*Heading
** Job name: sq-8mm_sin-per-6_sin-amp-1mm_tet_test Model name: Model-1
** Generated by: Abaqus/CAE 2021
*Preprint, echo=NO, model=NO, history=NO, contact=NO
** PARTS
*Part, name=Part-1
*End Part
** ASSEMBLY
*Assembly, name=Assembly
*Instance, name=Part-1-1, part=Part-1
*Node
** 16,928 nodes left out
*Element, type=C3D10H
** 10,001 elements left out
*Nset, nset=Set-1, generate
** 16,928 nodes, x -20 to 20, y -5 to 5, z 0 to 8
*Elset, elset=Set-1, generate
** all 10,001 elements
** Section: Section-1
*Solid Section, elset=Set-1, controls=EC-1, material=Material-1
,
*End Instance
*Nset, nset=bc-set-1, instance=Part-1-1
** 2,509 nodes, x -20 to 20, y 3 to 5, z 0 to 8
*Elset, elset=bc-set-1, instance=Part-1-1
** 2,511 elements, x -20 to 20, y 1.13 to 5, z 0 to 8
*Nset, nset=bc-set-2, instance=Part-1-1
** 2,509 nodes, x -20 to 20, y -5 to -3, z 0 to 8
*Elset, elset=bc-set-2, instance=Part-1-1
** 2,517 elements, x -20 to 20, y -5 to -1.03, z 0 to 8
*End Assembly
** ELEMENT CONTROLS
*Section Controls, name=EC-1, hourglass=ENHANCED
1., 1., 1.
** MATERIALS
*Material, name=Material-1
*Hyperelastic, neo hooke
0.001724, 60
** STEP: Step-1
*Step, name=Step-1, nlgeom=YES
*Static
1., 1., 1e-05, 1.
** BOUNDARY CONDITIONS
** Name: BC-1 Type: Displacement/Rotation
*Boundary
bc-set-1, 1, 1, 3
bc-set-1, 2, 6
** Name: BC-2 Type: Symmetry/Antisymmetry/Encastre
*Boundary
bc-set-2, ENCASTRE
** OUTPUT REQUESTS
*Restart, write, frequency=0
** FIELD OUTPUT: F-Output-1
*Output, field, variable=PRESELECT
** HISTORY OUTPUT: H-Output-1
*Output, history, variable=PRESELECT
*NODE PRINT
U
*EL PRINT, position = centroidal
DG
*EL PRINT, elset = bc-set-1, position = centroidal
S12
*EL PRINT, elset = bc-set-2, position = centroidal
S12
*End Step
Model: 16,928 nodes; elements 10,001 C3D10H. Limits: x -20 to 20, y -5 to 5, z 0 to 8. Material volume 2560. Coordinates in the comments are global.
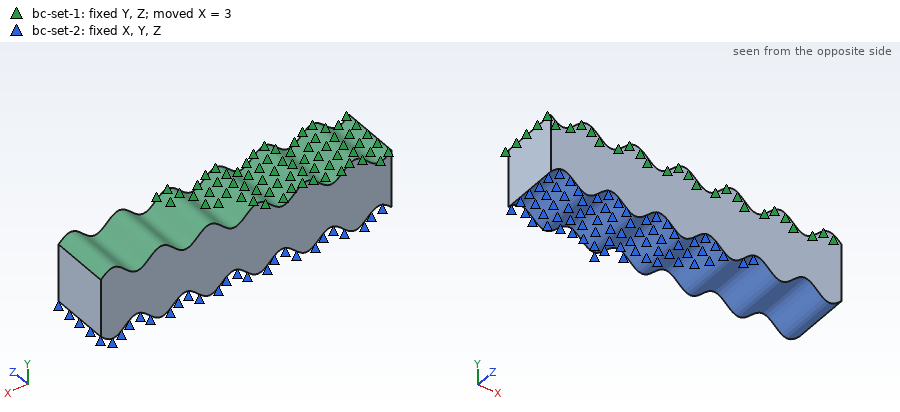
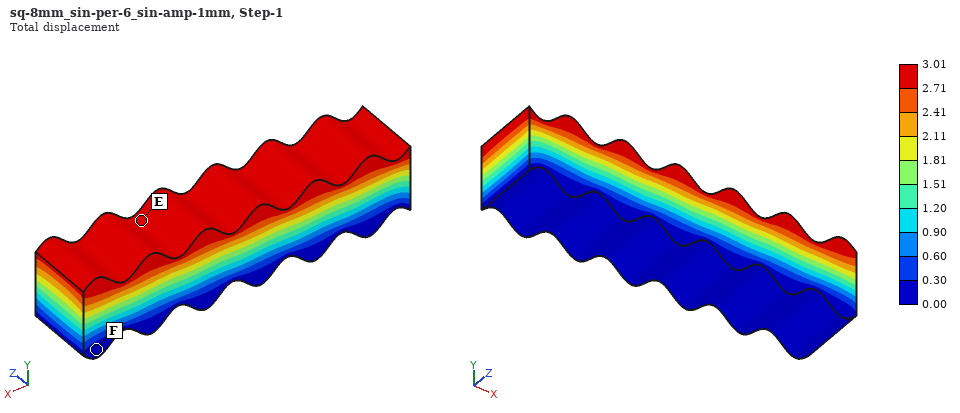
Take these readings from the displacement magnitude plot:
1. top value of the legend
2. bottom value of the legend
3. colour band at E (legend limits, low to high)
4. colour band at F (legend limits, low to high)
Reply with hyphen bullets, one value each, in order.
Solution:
- 3.01
- 0.00
- 2.71 to 3.01
- 0.00 to 0.30
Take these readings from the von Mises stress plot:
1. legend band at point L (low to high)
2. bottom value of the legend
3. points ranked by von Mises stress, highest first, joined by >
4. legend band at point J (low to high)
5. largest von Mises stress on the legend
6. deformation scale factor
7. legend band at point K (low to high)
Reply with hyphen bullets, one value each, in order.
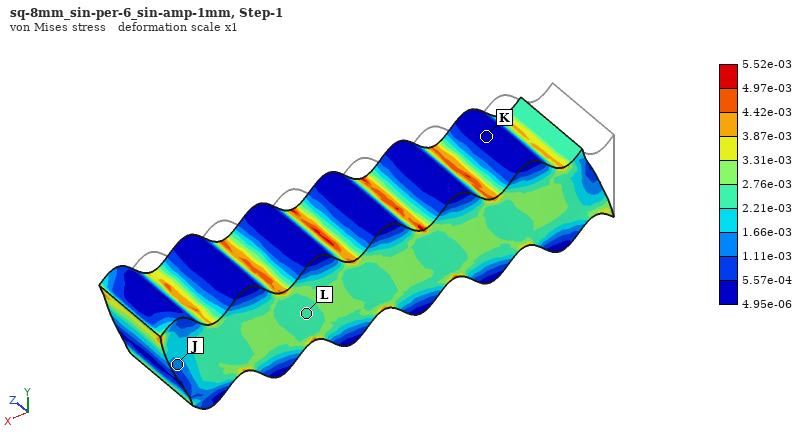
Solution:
- 2.21e-03 to 2.76e-03
- 4.95e-06
- L > J > K
- 1.11e-03 to 1.66e-03
- 5.52e-03
- 1
- 4.95e-06 to 5.57e-04
